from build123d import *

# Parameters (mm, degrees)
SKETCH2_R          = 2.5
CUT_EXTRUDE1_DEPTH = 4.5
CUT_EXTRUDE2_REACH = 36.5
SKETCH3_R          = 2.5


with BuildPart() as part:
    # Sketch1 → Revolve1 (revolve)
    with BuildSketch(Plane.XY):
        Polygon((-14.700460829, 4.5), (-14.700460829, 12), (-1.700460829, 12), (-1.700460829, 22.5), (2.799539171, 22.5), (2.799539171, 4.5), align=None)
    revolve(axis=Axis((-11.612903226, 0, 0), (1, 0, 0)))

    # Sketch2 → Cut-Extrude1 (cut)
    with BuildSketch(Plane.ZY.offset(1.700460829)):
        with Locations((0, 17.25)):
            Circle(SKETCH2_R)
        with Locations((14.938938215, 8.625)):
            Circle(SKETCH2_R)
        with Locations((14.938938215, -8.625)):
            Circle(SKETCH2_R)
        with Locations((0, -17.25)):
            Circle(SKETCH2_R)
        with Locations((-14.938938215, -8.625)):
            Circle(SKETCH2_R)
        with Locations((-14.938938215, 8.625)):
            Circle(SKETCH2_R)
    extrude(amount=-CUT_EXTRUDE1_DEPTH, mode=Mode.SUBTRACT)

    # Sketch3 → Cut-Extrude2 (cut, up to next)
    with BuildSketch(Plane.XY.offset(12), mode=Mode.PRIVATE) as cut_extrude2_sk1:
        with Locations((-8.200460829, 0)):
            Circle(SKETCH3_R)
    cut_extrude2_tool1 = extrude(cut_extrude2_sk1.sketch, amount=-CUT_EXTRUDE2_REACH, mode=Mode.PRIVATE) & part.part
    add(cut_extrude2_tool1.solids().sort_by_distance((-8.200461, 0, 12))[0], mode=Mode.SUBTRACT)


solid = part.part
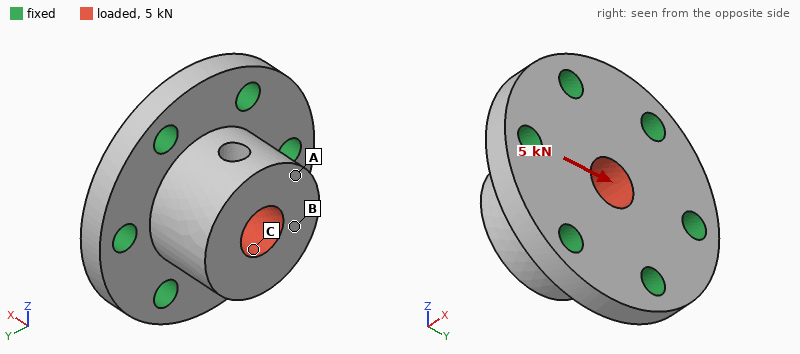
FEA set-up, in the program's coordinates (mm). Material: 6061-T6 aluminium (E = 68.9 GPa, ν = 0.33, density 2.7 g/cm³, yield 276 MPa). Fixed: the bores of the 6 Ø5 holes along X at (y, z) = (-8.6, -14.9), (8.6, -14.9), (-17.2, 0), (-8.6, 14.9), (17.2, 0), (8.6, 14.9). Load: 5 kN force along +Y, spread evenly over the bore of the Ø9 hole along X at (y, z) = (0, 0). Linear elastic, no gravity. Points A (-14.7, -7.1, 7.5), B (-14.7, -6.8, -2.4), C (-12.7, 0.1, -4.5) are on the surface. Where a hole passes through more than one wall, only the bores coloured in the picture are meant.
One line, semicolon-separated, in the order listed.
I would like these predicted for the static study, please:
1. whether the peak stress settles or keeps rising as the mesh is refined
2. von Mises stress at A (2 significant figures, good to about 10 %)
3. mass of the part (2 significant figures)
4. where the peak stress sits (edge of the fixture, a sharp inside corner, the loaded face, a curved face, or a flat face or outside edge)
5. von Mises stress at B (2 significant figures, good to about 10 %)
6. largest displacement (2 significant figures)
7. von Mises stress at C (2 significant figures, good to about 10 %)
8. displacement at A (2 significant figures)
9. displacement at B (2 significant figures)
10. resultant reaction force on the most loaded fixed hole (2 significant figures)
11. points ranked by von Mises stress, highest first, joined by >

keeps rising; 7.3 MPa; 30 g; edge of the fixture; 13 MPa; 13 µm; 24 MPa; 12 µm; 13 µm; 1.5 kN; C > B > A
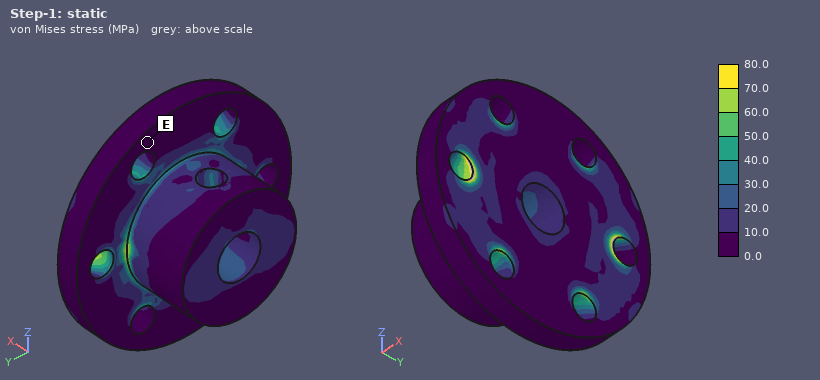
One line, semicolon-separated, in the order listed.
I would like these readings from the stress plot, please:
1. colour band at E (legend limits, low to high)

0.0 to 10.0 MPa
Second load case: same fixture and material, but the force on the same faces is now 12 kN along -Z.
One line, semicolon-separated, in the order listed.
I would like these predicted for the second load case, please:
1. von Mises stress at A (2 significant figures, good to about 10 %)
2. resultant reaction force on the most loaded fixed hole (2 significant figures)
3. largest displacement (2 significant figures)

20 MPa; 3.1 kN; 31 µm
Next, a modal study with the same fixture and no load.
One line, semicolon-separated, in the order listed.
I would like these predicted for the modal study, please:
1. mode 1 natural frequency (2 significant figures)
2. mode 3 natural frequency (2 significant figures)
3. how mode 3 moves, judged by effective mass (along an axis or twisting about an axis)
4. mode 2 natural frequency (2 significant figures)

27 kHz; 31 kHz; along X; 27 kHz
